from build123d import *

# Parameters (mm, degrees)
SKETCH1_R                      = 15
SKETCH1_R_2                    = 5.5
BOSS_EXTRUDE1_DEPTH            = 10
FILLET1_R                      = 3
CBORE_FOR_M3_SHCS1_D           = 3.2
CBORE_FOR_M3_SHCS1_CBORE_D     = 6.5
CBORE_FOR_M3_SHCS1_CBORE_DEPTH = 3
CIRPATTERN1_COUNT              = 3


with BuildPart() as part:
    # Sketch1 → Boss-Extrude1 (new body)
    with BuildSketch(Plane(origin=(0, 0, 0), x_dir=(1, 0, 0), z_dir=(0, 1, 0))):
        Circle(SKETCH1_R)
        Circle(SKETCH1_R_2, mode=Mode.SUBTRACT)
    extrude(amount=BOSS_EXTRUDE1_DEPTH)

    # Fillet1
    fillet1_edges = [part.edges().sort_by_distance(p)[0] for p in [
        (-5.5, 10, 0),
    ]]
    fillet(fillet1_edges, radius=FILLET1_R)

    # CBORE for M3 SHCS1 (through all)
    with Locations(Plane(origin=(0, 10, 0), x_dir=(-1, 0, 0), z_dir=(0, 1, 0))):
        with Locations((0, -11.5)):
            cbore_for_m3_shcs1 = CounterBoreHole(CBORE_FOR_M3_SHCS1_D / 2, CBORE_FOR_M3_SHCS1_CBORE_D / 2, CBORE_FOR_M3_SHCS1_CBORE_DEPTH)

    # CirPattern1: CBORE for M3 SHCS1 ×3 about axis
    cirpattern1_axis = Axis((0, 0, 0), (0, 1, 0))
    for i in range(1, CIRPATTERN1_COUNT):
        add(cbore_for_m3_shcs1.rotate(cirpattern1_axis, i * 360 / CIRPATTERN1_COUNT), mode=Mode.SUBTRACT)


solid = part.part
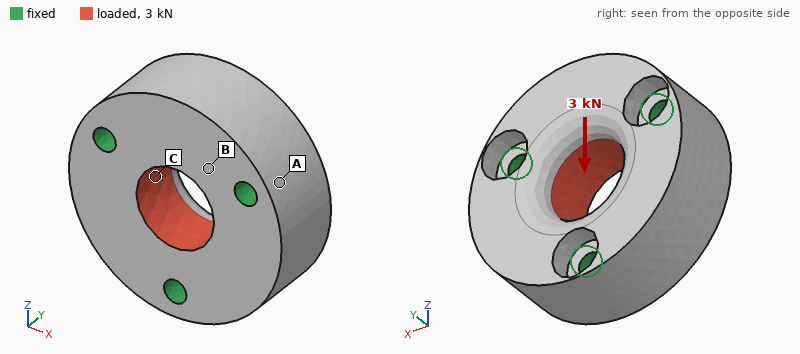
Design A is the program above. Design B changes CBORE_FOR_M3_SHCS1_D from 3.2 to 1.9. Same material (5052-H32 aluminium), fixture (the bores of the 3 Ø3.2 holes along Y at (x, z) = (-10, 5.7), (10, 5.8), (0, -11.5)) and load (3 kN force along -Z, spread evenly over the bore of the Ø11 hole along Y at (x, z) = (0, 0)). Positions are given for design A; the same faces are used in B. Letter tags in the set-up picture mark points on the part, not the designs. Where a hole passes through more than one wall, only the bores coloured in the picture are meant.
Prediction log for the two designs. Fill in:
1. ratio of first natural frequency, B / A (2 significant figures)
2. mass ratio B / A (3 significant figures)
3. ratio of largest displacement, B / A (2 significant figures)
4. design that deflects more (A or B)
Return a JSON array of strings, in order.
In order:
["0.86", "1.02", "1.2", "B"]
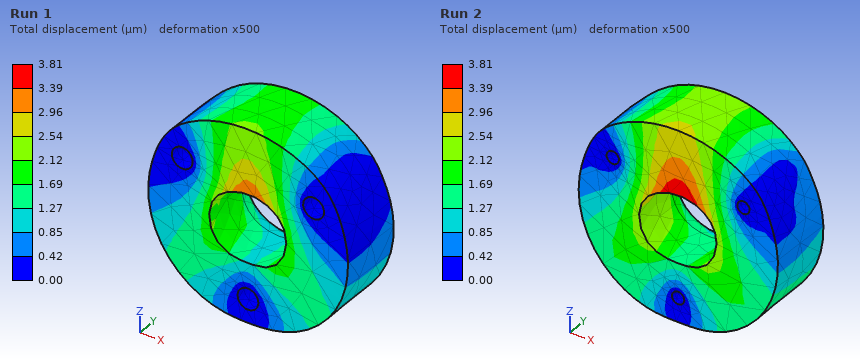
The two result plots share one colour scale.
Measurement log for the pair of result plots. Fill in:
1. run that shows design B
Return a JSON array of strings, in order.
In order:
["Run 2"]
